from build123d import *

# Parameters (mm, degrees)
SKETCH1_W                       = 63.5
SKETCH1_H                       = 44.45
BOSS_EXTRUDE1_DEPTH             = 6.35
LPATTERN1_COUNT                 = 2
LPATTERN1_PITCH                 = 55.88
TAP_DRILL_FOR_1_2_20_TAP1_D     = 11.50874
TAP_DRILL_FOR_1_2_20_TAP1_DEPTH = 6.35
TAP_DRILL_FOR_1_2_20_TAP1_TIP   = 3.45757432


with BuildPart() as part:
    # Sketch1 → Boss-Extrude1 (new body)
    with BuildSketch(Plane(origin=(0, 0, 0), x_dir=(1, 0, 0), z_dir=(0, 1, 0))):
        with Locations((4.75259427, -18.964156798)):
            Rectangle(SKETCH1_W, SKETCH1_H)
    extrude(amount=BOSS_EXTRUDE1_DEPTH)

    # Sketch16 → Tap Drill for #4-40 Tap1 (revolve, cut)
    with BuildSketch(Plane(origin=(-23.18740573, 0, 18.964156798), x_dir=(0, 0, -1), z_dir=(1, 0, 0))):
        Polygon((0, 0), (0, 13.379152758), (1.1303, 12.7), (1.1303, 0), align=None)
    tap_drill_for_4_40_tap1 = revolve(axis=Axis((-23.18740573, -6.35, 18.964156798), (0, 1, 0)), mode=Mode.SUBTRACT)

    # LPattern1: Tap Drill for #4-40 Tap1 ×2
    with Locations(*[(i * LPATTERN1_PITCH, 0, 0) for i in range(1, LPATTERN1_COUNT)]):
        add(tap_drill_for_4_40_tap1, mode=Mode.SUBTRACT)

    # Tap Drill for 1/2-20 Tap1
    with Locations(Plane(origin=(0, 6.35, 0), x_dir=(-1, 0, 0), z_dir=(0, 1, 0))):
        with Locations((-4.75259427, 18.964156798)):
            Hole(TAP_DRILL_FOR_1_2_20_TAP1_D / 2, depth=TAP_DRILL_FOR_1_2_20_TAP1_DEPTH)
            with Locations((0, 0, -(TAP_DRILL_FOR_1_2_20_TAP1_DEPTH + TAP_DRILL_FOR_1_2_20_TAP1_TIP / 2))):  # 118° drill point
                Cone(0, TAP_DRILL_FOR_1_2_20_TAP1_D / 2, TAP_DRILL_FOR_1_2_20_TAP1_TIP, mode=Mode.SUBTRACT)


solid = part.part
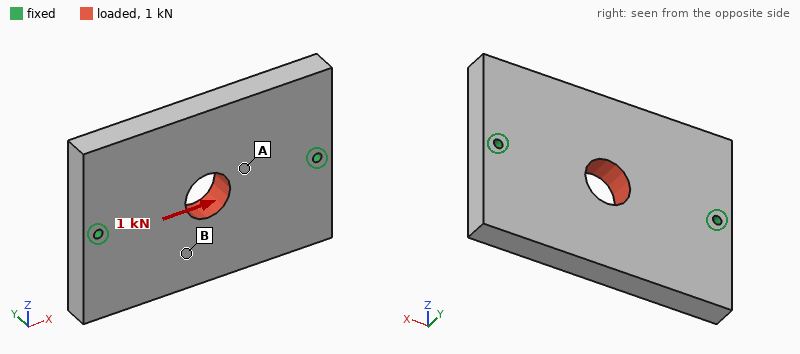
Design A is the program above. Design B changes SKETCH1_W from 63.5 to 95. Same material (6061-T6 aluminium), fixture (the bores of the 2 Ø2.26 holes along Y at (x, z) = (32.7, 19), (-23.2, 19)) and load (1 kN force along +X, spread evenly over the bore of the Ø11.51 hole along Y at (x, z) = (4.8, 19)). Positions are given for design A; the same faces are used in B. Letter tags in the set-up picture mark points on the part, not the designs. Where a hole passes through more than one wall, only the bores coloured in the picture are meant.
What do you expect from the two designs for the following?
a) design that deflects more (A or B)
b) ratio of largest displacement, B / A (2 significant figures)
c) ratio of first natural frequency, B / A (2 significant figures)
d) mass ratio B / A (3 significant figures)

A
0.85
0.97
1.52
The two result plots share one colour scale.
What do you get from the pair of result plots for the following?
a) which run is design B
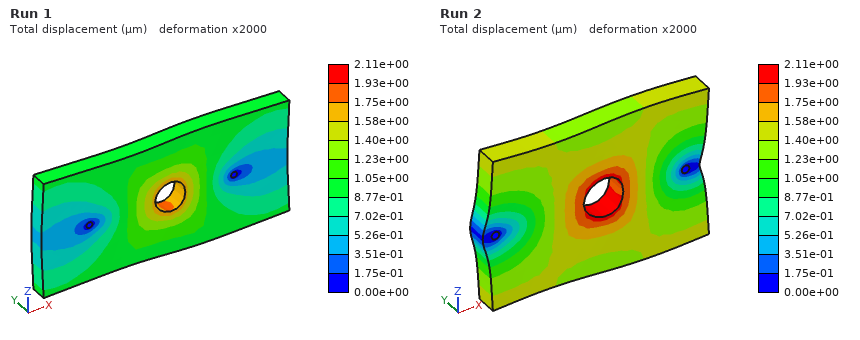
Run 1
